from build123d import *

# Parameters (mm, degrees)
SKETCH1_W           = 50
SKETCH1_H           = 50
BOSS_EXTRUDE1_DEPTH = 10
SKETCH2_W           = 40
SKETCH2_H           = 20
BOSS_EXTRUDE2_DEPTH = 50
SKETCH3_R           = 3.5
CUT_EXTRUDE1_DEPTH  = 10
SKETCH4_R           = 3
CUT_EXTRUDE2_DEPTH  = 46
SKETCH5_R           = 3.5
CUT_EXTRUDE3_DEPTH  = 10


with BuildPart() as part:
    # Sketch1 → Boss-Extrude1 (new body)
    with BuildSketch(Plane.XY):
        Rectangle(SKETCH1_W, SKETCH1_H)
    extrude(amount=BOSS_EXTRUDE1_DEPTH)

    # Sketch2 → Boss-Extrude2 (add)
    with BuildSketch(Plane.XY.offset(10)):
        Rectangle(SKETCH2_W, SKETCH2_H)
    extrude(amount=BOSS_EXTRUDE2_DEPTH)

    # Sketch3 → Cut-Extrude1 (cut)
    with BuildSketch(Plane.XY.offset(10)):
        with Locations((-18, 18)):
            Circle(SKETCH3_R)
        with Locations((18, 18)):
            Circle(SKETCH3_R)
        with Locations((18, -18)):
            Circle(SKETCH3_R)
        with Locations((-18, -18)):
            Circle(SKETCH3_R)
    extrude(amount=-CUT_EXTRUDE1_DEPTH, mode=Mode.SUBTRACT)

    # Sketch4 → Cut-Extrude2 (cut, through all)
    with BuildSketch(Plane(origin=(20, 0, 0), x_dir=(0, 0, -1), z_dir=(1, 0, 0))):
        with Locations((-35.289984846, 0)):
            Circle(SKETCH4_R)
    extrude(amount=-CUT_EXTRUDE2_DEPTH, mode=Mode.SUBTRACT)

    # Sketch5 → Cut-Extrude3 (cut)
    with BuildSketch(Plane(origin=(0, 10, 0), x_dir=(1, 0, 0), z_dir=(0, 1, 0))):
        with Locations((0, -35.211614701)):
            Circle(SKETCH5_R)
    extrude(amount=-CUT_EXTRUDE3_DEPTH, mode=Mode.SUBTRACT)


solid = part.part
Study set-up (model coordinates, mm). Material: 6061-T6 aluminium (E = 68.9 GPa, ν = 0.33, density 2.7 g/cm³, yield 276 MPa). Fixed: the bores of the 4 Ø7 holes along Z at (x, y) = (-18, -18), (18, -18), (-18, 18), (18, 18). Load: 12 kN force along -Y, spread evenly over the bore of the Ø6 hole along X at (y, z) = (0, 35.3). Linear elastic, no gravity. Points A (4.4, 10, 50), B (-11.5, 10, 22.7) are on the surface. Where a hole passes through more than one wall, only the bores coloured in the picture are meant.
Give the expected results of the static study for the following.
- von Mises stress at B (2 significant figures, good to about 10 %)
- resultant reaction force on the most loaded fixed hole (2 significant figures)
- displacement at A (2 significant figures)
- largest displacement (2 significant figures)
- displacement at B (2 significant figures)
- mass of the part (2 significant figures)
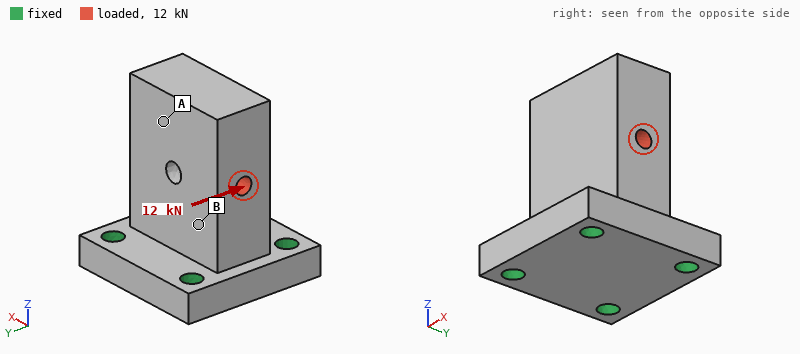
57 MPa
6.9 kN
0.16 mm
0.20 mm
0.058 mm
170 g
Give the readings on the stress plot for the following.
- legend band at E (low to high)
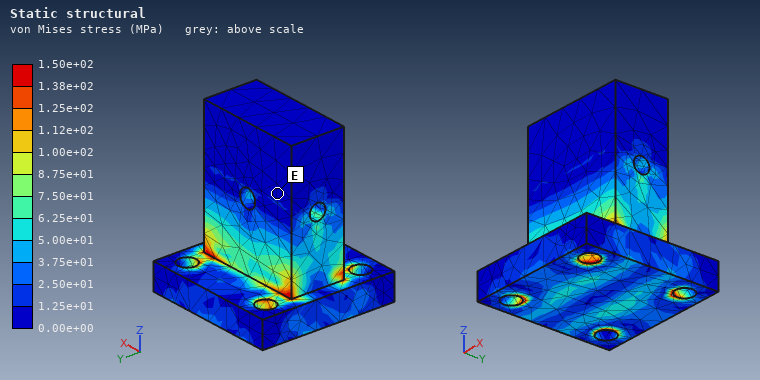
0.00e+00 to 1.25e+01 MPa
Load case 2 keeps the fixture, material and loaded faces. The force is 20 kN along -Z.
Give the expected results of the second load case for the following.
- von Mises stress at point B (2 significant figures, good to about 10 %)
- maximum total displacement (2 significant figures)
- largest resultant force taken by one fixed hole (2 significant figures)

24 MPa
29 µm
5.3 kN
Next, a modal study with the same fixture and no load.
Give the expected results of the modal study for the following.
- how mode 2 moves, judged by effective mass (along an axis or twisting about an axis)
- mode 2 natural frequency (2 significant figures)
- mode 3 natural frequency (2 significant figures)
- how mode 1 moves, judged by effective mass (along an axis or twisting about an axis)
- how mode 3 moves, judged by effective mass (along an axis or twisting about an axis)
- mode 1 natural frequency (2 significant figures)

along X
6100 Hz
11 kHz
along Y
twisting about Z
4500 Hz
